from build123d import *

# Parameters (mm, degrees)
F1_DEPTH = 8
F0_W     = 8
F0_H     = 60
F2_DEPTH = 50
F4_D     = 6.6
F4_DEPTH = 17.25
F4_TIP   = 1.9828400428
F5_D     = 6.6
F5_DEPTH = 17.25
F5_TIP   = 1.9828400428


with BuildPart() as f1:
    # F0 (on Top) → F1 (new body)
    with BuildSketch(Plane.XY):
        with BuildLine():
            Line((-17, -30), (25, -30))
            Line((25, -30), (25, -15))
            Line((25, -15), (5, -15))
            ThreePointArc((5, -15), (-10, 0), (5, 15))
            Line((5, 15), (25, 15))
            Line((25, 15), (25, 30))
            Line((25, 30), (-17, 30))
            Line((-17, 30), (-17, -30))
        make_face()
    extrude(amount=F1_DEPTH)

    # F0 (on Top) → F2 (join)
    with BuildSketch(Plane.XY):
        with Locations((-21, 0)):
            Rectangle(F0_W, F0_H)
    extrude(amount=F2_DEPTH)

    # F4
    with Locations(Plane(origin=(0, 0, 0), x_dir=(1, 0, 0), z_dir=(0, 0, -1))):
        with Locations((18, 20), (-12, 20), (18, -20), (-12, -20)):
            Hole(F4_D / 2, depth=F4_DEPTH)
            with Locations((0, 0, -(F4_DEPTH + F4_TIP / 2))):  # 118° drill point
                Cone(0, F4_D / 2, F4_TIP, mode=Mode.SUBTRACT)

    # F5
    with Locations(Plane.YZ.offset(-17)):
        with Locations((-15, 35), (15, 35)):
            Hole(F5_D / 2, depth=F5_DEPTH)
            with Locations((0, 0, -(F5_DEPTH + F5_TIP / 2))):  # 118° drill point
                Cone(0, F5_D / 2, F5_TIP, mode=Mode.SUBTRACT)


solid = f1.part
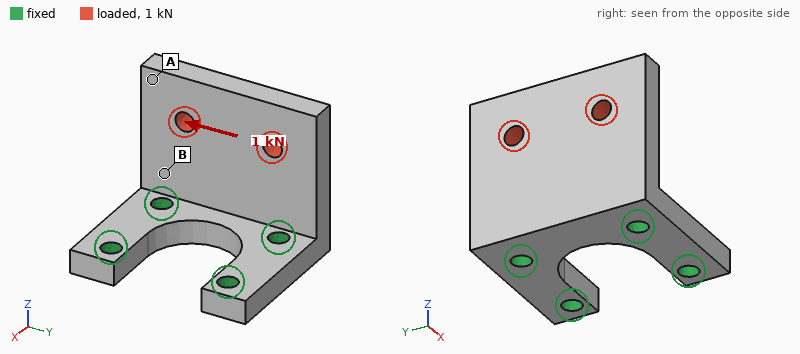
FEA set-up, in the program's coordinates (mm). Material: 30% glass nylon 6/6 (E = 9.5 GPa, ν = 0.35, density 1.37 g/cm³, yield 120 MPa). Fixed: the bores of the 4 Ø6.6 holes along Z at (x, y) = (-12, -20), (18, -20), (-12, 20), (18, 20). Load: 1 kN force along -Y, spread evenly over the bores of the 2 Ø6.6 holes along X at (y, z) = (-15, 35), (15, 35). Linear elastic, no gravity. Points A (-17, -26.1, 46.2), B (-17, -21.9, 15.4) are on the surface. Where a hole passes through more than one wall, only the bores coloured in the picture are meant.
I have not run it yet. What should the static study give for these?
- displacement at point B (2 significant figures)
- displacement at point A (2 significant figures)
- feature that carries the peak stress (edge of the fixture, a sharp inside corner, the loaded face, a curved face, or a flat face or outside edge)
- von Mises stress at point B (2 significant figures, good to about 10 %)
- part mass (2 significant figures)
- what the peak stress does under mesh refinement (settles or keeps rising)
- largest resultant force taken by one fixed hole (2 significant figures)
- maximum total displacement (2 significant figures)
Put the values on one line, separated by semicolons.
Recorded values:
33 µm; 89 µm; edge of the fixture; 7.8 MPa; 48 g; keeps rising; 880 N; 97 µm
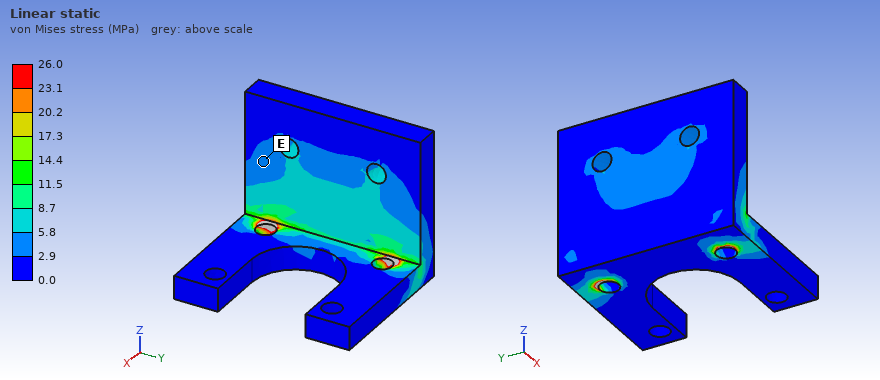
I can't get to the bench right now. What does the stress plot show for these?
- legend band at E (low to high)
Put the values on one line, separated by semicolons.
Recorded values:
2.9 to 5.8 MPa
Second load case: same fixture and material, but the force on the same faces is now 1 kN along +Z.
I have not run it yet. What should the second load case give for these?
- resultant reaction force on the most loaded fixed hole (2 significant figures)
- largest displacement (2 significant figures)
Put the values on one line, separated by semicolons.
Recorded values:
520 N; 0.10 mm
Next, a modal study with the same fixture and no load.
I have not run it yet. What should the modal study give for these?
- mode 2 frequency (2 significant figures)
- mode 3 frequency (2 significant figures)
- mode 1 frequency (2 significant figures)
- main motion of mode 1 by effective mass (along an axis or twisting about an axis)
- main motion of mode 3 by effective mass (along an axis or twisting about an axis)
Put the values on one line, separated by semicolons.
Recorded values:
2700 Hz; 4500 Hz; 1300 Hz; along X; along Y
